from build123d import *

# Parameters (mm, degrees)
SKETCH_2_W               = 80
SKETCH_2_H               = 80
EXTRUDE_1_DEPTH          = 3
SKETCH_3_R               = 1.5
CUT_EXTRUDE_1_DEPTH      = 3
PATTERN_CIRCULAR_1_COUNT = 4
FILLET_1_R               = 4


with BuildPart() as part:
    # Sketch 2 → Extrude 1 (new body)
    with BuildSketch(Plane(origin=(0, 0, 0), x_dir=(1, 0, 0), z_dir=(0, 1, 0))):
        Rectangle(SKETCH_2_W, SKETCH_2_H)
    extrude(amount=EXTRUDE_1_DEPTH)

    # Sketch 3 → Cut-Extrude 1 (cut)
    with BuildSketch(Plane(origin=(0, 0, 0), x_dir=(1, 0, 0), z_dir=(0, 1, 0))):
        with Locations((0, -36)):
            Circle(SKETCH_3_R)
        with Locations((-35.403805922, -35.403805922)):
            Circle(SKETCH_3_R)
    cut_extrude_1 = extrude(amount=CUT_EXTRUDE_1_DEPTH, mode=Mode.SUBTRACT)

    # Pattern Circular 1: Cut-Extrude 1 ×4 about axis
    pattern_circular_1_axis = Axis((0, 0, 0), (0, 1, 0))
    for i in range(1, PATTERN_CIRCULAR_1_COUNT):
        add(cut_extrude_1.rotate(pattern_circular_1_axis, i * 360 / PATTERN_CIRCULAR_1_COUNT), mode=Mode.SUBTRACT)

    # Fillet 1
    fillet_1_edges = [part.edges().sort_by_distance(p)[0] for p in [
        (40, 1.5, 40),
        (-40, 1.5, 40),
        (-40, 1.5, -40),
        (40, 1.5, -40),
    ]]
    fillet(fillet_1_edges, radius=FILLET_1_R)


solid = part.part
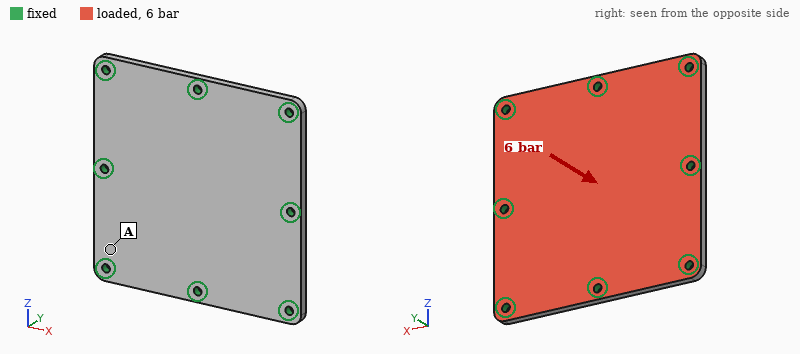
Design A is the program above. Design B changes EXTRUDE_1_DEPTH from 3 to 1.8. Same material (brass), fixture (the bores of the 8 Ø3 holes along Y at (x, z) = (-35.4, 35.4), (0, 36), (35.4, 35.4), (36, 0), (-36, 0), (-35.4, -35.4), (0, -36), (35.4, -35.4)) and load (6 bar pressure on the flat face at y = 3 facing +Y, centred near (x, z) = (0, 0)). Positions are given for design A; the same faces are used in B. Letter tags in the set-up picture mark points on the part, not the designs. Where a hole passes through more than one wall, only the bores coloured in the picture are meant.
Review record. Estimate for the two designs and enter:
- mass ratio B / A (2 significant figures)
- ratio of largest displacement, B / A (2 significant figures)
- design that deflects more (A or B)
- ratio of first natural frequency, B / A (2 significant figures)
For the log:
0.60
4.3
B
0.63
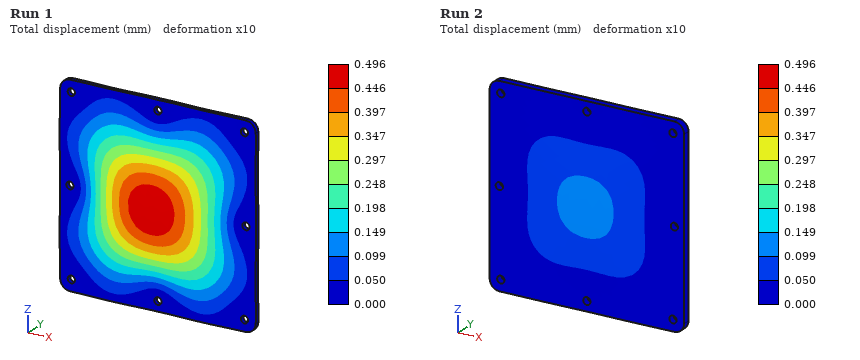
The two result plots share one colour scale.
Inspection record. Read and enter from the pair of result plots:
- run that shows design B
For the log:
Run 1
